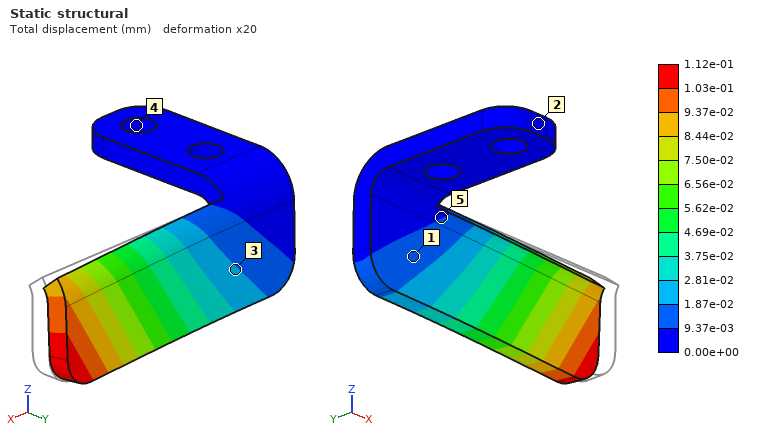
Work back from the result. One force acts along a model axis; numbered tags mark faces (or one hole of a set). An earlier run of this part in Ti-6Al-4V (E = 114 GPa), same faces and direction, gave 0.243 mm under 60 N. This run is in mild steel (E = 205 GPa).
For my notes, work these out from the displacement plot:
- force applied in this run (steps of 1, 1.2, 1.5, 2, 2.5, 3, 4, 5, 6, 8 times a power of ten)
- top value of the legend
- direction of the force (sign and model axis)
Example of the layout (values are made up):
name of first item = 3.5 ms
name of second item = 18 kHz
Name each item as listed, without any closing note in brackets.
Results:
force applied in this run = 50 N
top value of the legend = 1.12e-01 mm
direction of the force = +Y
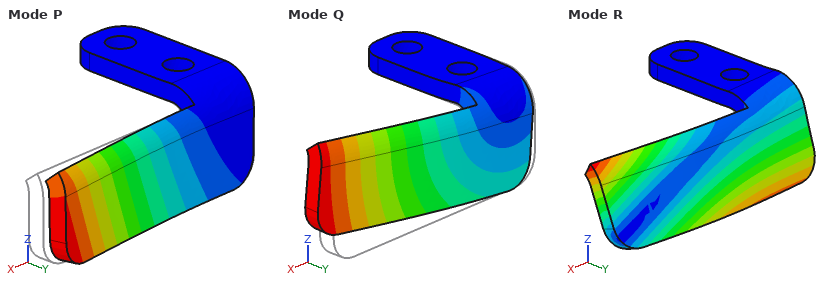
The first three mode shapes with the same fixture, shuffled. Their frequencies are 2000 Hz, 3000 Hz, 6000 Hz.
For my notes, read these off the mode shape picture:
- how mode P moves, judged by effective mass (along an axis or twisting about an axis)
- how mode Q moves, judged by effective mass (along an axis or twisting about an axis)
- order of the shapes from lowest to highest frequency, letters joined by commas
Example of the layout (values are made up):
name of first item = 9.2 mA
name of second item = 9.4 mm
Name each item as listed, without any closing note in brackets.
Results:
how mode P moves, judged by effective mass = along Y
how mode Q moves, judged by effective mass = along Z
order of the shapes from lowest to highest frequency, letters joined by commas = P, Q, R
